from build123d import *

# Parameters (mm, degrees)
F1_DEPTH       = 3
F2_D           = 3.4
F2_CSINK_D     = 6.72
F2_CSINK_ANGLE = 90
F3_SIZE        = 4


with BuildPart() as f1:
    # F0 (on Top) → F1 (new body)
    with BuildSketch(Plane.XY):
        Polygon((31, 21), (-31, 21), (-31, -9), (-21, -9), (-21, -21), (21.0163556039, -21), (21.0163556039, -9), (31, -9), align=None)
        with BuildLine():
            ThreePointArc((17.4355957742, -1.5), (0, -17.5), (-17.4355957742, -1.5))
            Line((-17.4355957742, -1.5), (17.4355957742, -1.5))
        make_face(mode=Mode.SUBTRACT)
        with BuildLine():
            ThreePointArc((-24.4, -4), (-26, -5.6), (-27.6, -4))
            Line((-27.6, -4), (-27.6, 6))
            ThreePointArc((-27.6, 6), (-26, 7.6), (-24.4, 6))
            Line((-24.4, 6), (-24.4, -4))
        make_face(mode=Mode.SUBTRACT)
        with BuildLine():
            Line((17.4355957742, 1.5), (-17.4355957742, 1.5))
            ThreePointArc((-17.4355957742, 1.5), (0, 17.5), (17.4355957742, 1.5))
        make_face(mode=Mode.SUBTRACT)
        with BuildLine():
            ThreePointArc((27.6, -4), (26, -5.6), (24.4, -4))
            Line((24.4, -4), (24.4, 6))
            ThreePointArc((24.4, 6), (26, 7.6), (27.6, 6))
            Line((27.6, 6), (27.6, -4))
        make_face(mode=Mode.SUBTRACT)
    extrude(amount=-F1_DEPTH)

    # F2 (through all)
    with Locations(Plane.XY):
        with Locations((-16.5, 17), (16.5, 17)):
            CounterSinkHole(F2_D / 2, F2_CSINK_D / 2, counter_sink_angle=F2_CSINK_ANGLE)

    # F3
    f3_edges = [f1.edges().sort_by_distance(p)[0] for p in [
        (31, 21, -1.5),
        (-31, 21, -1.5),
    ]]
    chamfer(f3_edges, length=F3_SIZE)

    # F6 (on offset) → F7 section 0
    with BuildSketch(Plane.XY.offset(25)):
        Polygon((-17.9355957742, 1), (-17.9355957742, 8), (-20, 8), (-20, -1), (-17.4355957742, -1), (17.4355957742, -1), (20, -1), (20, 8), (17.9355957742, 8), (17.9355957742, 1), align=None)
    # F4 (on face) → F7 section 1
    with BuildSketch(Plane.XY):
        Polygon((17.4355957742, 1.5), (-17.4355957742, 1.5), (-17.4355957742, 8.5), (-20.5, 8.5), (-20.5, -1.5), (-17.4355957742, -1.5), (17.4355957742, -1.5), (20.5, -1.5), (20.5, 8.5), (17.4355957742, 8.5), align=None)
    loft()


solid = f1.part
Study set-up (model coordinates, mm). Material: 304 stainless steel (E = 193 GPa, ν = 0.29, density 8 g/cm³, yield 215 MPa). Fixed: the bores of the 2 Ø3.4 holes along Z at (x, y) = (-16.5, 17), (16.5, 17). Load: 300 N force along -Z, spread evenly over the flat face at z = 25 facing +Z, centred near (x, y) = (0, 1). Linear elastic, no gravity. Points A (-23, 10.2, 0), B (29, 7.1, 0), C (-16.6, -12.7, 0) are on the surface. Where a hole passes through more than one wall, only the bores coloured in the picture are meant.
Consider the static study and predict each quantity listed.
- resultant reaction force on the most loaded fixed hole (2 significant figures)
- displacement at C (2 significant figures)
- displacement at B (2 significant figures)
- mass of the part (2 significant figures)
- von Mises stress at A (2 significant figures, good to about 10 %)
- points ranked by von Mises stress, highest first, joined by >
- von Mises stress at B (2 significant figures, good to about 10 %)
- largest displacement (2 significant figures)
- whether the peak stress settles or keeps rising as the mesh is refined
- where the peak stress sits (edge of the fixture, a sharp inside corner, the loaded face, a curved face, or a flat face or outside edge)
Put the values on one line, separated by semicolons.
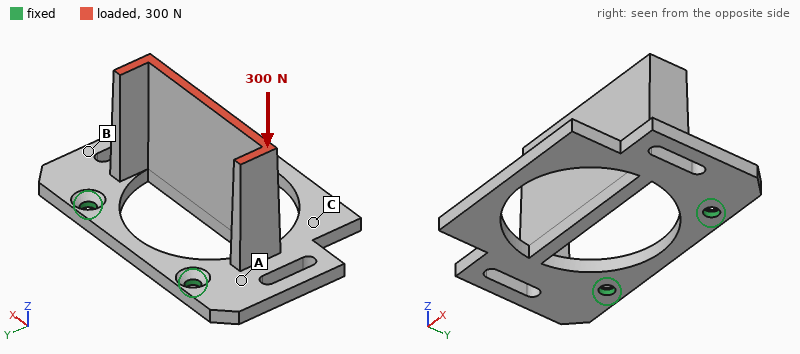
150 N; 0.12 mm; 0.032 mm; 61 g; 57 MPa; A > B > C; 32 MPa; 0.16 mm; keeps rising; edge of the fixture
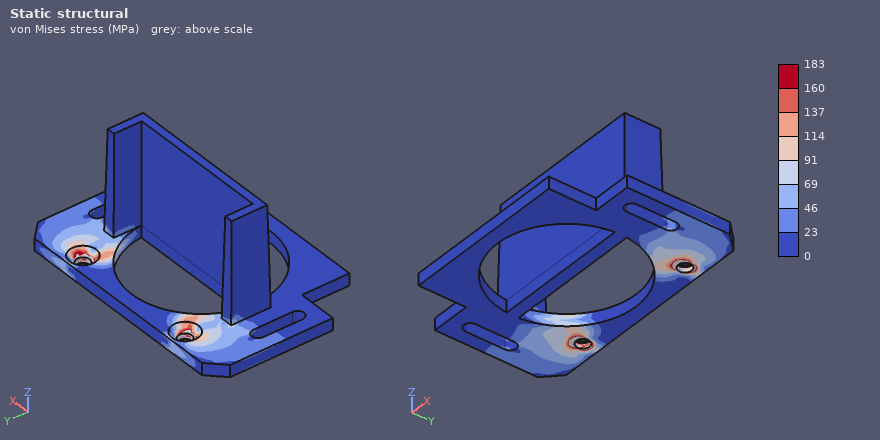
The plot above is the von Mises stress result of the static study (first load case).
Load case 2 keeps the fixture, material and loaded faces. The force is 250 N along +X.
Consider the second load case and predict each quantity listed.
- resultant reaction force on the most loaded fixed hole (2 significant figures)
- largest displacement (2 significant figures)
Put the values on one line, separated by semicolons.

220 N; 68 µm
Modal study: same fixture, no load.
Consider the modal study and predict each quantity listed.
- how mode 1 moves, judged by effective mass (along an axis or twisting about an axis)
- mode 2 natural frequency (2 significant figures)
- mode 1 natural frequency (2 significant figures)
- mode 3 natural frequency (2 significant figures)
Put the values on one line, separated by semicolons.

along Z; 2200 Hz; 970 Hz; 3800 Hz
